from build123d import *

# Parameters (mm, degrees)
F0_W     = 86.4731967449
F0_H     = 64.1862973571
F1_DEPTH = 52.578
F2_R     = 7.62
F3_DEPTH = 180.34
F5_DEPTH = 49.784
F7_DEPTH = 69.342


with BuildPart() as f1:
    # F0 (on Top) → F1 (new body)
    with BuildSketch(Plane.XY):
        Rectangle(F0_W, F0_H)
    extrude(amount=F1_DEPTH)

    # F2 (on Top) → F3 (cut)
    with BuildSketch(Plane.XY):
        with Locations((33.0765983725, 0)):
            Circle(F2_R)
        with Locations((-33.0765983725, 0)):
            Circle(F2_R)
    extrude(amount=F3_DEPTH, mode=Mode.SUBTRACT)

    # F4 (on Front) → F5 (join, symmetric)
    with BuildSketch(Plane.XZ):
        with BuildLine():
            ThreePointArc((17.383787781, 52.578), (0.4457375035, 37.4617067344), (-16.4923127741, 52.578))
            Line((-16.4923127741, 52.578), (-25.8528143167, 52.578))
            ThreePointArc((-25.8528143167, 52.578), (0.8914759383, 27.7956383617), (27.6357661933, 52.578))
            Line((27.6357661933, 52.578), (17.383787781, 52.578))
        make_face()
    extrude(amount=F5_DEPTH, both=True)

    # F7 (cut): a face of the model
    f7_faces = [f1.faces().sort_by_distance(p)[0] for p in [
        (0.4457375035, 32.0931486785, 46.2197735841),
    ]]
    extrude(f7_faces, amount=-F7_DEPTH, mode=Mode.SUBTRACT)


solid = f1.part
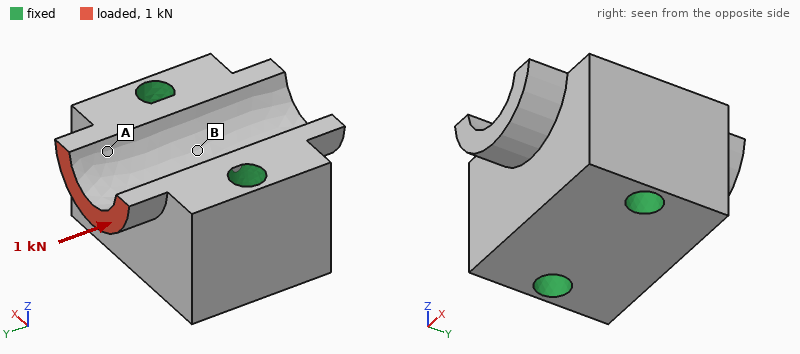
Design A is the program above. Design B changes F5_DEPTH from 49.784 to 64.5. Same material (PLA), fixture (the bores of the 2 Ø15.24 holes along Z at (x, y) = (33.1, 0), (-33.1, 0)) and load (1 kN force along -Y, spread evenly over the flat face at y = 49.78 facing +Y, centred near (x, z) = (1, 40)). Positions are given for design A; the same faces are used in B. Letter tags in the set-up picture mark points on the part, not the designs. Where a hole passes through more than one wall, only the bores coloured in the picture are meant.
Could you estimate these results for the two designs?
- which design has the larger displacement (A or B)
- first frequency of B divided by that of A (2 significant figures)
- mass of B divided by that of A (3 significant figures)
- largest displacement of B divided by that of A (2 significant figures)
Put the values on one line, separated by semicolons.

B; 0.58; 1.07; 1.2
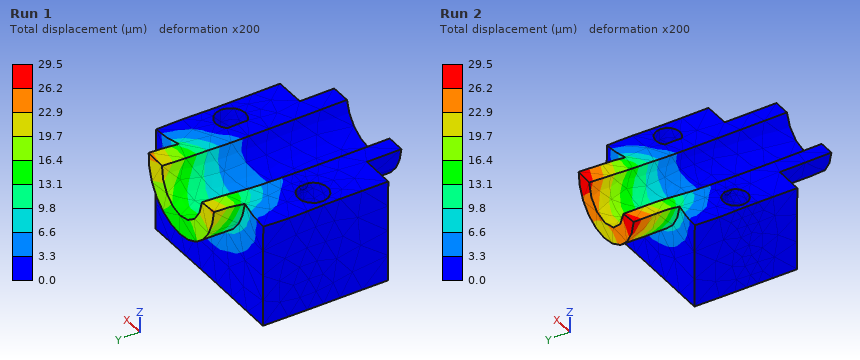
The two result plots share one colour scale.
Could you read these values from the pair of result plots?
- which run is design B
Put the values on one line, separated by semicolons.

Run 2
